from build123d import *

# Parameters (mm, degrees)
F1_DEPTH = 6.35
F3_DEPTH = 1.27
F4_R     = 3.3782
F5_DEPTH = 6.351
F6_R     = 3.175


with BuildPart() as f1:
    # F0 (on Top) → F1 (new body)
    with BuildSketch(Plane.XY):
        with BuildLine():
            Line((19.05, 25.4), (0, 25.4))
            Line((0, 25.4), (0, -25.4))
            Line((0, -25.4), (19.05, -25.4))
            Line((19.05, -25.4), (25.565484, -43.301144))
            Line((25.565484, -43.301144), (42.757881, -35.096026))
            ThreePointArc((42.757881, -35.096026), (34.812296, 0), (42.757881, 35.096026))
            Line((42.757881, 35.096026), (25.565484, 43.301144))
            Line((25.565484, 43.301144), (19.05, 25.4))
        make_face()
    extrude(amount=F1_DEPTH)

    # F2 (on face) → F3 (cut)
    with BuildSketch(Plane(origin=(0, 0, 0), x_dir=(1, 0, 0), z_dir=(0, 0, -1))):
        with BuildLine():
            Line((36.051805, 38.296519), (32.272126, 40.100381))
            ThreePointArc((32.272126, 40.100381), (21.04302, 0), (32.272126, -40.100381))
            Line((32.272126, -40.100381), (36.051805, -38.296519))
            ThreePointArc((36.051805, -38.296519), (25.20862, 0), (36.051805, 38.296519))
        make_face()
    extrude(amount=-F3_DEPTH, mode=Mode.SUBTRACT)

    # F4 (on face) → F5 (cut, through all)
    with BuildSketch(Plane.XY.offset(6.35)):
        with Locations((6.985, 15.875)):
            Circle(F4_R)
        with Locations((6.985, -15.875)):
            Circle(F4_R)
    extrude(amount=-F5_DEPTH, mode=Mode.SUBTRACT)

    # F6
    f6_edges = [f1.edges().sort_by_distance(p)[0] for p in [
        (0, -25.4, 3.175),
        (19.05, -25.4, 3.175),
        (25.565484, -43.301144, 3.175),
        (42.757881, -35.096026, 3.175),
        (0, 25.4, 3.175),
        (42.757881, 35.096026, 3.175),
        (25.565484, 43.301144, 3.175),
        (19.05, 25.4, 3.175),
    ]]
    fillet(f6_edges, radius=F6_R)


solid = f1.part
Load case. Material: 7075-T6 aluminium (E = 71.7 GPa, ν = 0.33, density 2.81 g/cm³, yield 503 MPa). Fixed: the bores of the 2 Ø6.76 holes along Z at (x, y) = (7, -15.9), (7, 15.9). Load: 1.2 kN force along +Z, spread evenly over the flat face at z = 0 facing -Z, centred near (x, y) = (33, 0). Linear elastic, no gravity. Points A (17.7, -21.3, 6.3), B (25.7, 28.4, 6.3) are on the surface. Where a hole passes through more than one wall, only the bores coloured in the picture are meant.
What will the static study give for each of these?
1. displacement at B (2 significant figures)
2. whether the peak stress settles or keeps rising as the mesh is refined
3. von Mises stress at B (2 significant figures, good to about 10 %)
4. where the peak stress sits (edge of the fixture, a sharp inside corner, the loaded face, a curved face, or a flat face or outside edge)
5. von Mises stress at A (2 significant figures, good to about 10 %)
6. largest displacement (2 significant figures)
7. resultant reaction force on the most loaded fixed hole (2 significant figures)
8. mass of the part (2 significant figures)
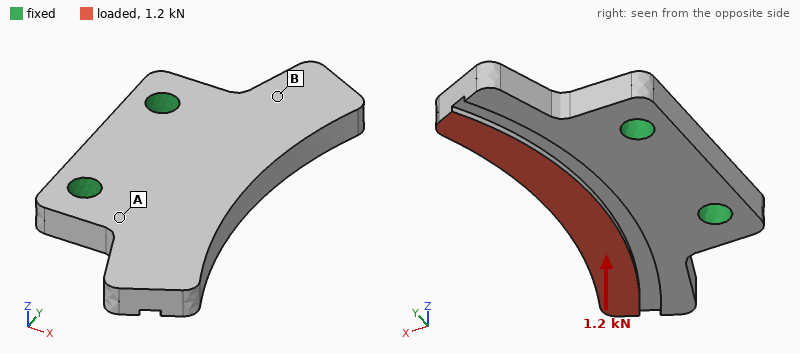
0.058 mm
keeps rising
20 MPa
edge of the fixture
57 MPa
0.15 mm
600 N
40 g
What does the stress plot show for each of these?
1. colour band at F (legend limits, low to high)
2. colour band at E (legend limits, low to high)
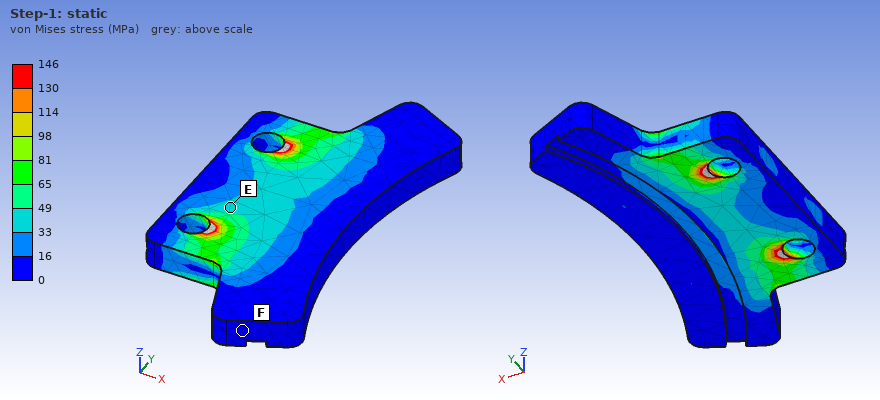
0 to 16 MPa
33 to 49 MPa
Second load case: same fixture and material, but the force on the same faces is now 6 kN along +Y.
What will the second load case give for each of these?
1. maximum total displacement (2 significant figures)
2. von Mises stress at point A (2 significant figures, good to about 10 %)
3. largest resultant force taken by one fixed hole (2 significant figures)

0.13 mm
56 MPa
5.1 kN
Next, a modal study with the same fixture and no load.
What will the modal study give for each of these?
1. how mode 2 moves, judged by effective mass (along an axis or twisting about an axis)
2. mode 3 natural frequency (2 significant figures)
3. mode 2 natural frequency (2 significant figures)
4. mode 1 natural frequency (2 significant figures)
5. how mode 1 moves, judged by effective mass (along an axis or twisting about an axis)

twisting about X
8100 Hz
4400 Hz
4200 Hz
along Z
